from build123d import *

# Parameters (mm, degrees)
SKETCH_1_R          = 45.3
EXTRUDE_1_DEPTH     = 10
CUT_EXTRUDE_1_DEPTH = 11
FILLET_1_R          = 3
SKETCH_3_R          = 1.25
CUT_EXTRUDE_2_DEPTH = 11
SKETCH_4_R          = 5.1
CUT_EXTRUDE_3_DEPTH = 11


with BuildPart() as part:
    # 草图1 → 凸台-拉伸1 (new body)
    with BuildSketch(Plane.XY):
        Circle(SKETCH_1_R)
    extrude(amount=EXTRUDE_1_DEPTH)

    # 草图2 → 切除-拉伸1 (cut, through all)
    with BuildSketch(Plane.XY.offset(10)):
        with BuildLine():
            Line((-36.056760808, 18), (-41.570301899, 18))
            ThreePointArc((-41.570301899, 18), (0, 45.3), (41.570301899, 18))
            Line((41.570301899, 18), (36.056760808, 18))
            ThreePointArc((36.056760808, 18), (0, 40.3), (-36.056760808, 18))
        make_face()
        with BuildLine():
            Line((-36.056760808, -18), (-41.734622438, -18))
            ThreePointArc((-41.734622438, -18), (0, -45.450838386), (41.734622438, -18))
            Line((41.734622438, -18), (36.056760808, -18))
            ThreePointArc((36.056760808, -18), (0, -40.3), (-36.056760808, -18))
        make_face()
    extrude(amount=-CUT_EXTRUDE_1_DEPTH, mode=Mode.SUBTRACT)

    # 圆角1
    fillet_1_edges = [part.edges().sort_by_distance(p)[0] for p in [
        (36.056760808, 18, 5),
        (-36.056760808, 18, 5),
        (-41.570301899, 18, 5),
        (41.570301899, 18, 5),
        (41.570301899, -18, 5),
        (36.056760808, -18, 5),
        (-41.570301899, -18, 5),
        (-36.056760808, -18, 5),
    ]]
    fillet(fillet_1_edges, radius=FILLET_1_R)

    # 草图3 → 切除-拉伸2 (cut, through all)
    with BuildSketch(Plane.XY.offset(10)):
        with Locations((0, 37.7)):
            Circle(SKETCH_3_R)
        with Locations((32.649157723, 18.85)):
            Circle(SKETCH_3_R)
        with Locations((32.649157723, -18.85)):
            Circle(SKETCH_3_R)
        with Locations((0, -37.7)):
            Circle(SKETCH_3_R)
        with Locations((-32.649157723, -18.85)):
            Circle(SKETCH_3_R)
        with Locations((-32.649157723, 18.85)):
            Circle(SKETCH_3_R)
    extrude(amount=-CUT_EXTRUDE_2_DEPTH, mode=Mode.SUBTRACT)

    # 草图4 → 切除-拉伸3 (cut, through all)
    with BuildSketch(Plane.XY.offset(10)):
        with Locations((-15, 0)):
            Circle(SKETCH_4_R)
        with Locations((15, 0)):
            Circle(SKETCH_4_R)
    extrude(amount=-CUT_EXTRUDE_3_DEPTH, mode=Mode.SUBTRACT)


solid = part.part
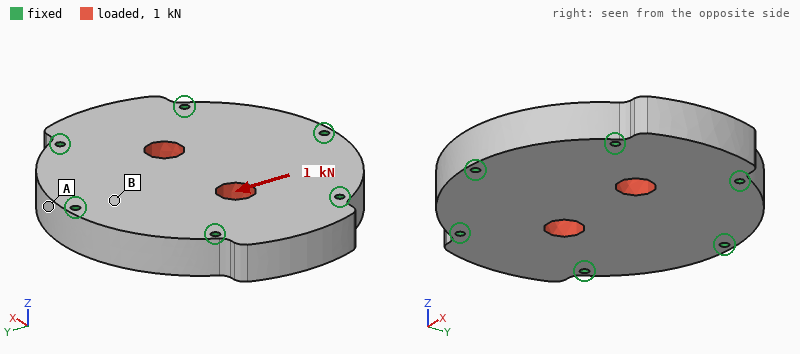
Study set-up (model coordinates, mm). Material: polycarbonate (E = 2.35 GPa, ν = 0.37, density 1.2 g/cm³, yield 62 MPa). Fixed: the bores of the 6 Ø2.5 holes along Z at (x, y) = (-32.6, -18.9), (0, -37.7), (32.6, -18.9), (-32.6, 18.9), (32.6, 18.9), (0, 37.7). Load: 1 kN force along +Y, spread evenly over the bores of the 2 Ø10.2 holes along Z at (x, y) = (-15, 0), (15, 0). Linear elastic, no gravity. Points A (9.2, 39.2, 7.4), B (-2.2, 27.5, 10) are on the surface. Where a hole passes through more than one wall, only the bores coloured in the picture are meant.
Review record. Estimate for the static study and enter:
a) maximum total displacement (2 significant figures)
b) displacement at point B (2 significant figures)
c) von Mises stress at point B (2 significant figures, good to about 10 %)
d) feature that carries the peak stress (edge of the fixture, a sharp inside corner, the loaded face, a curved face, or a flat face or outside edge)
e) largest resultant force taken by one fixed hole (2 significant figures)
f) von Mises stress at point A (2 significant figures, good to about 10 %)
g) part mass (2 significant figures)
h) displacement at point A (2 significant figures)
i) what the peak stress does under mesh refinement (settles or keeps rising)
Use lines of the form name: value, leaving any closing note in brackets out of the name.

maximum total displacement: 20 µm
displacement at point B: 8.6 µm
von Mises stress at point B: 1.4 MPa
feature that carries the peak stress: edge of the fixture
largest resultant force taken by one fixed hole: 200 N
von Mises stress at point A: 0.59 MPa
part mass: 63 g
displacement at point A: 8.4 µm
what the peak stress does under mesh refinement: keeps rising
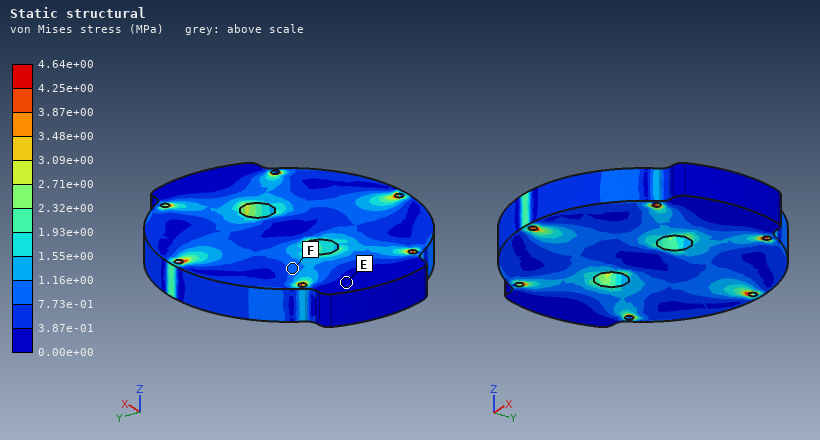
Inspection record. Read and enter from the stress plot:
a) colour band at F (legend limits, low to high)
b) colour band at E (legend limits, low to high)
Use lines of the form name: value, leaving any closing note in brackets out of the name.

colour band at F: 7.73e-01 to 1.16e+00 MPa
colour band at E: 0.00e+00 to 3.87e-01 MPa
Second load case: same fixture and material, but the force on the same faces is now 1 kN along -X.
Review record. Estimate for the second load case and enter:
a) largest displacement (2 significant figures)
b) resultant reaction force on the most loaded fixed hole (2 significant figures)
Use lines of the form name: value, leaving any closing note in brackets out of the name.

largest displacement: 25 µm
resultant reaction force on the most loaded fixed hole: 220 N
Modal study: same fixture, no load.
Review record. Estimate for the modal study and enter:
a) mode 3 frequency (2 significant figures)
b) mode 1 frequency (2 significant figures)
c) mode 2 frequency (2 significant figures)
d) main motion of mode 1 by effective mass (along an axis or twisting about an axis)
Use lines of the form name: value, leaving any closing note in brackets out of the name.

mode 3 frequency: 5400 Hz
mode 1 frequency: 2900 Hz
mode 2 frequency: 5300 Hz
main motion of mode 1 by effective mass: along Z
